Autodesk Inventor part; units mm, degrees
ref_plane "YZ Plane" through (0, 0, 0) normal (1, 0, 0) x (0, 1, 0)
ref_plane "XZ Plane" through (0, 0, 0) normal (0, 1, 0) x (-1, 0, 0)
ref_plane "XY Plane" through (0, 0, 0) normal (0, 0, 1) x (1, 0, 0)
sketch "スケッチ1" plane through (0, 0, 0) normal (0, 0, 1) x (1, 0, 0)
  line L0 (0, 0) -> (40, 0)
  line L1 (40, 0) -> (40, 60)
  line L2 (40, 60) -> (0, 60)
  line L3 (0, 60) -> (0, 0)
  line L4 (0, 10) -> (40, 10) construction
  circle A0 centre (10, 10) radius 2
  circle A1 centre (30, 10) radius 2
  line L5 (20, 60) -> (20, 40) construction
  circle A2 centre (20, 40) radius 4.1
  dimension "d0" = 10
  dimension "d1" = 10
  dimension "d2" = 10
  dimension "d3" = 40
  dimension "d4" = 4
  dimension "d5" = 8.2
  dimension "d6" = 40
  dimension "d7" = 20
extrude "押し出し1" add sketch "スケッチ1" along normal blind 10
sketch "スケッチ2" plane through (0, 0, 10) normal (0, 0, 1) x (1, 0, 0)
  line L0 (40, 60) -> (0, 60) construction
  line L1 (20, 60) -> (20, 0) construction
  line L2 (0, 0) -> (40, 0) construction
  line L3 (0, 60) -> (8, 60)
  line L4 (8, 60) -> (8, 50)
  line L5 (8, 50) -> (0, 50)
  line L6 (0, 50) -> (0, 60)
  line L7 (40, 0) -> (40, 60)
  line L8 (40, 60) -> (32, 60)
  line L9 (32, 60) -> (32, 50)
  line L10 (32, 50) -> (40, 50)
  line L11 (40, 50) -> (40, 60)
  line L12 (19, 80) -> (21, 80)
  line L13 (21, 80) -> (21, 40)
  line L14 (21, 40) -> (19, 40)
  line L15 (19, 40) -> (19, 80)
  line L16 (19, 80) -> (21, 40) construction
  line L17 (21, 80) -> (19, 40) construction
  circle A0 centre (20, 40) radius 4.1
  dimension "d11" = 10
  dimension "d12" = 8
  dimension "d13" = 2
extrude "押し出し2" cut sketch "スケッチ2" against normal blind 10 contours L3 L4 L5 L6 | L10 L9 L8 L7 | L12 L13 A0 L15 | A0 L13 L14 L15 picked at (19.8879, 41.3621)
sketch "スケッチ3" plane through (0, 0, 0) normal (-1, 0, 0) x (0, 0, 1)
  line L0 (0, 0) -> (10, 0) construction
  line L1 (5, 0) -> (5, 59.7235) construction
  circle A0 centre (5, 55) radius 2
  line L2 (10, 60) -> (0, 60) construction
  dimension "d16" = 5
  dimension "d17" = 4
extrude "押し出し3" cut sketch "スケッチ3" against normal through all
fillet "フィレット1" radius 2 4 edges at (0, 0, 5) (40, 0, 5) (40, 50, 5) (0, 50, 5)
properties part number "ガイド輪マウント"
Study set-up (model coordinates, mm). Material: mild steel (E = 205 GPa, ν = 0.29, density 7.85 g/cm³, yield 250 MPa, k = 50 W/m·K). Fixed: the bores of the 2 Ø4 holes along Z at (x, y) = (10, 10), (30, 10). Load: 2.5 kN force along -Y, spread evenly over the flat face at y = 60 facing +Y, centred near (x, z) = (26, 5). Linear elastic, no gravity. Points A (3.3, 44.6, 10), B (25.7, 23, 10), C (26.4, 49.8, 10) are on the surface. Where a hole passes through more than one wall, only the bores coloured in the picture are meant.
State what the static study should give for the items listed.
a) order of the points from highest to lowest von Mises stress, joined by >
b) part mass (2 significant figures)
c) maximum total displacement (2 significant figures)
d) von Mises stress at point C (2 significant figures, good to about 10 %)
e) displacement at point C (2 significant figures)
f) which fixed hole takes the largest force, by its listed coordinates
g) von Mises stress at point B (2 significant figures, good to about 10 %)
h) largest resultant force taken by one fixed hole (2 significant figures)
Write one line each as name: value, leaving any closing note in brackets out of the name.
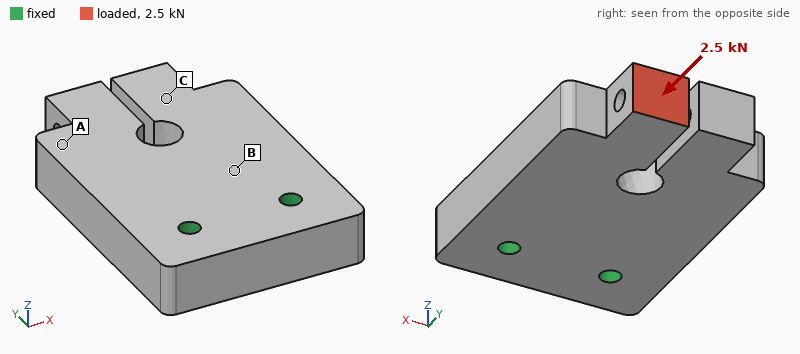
order of the points from highest to lowest von Mises stress, joined by >: C > B > A
part mass: 160 g
maximum total displacement: 9.3 µm
von Mises stress at point C: 35 MPa
displacement at point C: 4.6 µm
which fixed hole takes the largest force, by its listed coordinates: (30, 10)
von Mises stress at point B: 14 MPa
largest resultant force taken by one fixed hole: 2.0 kN
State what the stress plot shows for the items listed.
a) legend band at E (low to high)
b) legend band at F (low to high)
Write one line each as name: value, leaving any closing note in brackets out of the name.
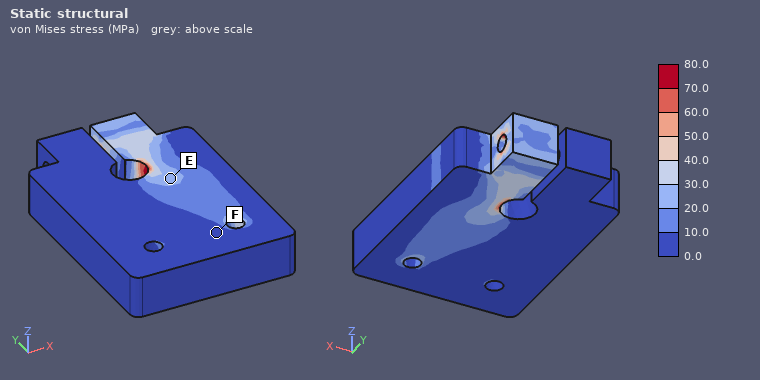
legend band at E: 20.0 to 30.0 MPa
legend band at F: 0.0 to 10.0 MPa
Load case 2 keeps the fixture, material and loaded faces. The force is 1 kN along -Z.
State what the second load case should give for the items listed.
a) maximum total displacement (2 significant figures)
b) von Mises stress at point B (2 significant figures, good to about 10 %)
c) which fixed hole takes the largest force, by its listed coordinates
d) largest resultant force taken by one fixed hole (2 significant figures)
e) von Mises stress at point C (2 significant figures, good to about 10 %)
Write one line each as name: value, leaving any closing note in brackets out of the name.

maximum total displacement: 0.11 mm
von Mises stress at point B: 69 MPa
which fixed hole takes the largest force, by its listed coordinates: (30, 10)
largest resultant force taken by one fixed hole: 710 N
von Mises stress at point C: 60 MPa
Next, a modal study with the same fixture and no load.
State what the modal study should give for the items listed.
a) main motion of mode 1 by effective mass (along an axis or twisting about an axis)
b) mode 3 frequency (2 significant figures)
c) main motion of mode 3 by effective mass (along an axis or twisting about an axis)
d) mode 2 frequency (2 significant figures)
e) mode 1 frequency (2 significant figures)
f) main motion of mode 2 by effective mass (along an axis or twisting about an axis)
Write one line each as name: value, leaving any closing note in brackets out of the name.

main motion of mode 1 by effective mass: along Z
mode 3 frequency: 8800 Hz
main motion of mode 3 by effective mass: along X
mode 2 frequency: 6600 Hz
mode 1 frequency: 3700 Hz
main motion of mode 2 by effective mass: twisting about Y
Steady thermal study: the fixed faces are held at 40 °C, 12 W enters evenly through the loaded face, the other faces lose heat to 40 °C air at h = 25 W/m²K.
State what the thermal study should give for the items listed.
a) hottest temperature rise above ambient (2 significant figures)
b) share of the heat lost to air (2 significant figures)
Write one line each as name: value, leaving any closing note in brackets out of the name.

hottest temperature rise above ambient: 71 K
share of the heat lost to air: 18 %
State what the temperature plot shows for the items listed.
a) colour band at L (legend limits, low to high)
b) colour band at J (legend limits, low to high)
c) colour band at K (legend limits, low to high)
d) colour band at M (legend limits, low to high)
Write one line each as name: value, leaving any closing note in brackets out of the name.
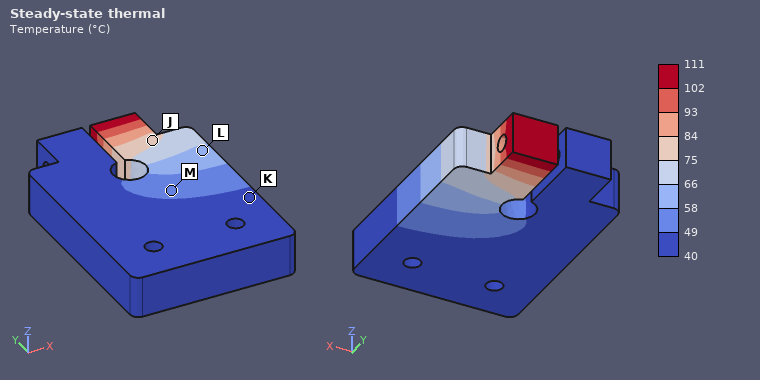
colour band at L: 58 to 66 °C
colour band at J: 75 to 84 °C
colour band at K: 40 to 49 °C
colour band at M: 49 to 58 °C
